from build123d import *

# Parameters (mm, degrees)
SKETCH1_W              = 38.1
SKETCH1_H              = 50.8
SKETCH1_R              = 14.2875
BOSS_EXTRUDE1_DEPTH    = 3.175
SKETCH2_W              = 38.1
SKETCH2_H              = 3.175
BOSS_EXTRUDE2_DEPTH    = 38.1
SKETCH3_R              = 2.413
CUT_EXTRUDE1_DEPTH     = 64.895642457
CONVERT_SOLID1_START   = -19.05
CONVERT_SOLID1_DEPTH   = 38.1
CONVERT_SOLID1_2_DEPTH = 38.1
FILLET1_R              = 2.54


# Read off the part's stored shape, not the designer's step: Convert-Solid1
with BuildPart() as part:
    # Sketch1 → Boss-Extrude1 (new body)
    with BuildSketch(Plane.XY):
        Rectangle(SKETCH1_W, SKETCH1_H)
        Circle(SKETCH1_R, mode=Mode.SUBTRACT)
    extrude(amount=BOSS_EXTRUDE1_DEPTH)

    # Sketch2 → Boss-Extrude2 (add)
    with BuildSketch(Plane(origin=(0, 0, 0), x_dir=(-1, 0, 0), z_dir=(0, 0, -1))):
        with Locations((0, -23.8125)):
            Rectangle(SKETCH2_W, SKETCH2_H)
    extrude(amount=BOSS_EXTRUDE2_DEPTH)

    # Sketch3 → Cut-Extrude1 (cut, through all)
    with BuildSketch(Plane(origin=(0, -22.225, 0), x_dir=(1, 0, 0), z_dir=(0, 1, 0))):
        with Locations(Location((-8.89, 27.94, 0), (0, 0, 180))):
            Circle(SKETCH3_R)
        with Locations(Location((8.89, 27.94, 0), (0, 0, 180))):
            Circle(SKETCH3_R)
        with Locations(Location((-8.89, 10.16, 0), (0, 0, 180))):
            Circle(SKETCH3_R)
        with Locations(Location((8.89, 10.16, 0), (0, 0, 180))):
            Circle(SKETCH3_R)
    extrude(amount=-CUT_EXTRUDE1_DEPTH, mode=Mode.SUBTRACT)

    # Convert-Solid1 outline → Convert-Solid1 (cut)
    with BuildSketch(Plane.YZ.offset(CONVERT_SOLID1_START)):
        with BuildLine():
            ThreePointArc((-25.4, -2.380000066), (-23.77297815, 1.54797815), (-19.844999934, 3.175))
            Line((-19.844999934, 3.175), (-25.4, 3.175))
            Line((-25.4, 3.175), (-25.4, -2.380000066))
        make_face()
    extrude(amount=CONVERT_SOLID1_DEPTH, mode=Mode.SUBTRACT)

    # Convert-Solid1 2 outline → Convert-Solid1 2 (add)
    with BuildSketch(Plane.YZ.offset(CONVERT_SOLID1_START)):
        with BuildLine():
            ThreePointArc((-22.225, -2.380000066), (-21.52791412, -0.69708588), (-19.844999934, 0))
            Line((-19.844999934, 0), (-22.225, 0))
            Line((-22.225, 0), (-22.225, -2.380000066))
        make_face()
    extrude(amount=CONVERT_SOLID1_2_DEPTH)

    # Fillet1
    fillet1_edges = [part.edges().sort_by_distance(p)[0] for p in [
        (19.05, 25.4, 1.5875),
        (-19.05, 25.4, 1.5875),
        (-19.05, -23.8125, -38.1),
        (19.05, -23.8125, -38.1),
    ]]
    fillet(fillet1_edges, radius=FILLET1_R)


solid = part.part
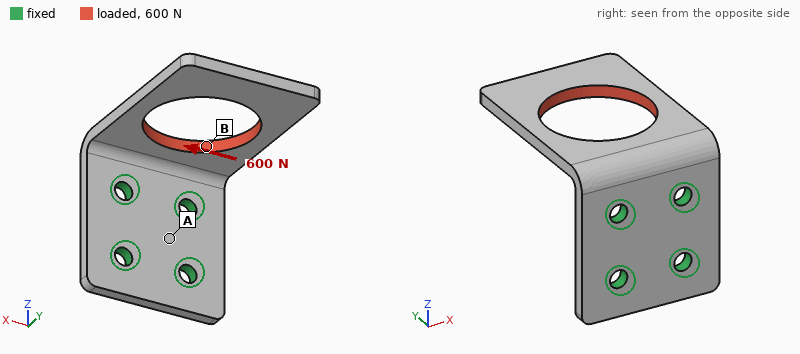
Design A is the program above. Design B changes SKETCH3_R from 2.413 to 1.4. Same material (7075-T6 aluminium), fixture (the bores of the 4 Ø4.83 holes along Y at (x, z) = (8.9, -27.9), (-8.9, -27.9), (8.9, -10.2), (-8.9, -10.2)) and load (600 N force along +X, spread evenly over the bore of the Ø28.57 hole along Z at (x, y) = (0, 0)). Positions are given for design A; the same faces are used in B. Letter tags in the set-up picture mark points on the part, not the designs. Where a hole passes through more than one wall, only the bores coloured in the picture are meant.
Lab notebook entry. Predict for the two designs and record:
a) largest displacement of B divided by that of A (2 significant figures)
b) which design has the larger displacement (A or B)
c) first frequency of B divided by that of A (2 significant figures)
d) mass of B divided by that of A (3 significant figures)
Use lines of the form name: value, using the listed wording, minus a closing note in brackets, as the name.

largest displacement of B divided by that of A: 1.2
which design has the larger displacement: B
first frequency of B divided by that of A: 0.98
mass of B divided by that of A: 1.02
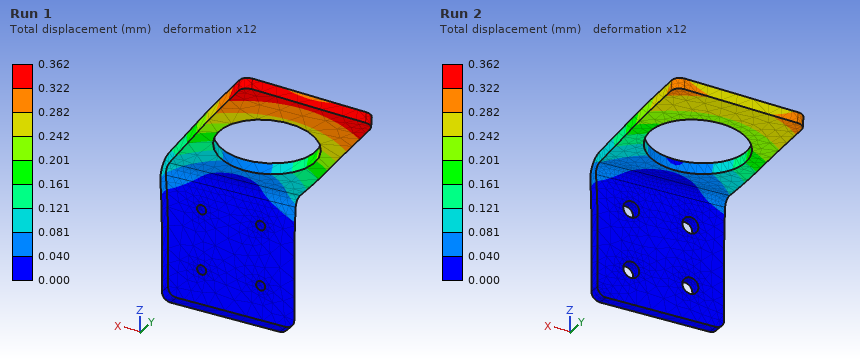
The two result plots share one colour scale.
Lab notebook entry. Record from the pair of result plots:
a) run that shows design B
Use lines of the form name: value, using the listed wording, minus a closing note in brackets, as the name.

run that shows design B: Run 1
